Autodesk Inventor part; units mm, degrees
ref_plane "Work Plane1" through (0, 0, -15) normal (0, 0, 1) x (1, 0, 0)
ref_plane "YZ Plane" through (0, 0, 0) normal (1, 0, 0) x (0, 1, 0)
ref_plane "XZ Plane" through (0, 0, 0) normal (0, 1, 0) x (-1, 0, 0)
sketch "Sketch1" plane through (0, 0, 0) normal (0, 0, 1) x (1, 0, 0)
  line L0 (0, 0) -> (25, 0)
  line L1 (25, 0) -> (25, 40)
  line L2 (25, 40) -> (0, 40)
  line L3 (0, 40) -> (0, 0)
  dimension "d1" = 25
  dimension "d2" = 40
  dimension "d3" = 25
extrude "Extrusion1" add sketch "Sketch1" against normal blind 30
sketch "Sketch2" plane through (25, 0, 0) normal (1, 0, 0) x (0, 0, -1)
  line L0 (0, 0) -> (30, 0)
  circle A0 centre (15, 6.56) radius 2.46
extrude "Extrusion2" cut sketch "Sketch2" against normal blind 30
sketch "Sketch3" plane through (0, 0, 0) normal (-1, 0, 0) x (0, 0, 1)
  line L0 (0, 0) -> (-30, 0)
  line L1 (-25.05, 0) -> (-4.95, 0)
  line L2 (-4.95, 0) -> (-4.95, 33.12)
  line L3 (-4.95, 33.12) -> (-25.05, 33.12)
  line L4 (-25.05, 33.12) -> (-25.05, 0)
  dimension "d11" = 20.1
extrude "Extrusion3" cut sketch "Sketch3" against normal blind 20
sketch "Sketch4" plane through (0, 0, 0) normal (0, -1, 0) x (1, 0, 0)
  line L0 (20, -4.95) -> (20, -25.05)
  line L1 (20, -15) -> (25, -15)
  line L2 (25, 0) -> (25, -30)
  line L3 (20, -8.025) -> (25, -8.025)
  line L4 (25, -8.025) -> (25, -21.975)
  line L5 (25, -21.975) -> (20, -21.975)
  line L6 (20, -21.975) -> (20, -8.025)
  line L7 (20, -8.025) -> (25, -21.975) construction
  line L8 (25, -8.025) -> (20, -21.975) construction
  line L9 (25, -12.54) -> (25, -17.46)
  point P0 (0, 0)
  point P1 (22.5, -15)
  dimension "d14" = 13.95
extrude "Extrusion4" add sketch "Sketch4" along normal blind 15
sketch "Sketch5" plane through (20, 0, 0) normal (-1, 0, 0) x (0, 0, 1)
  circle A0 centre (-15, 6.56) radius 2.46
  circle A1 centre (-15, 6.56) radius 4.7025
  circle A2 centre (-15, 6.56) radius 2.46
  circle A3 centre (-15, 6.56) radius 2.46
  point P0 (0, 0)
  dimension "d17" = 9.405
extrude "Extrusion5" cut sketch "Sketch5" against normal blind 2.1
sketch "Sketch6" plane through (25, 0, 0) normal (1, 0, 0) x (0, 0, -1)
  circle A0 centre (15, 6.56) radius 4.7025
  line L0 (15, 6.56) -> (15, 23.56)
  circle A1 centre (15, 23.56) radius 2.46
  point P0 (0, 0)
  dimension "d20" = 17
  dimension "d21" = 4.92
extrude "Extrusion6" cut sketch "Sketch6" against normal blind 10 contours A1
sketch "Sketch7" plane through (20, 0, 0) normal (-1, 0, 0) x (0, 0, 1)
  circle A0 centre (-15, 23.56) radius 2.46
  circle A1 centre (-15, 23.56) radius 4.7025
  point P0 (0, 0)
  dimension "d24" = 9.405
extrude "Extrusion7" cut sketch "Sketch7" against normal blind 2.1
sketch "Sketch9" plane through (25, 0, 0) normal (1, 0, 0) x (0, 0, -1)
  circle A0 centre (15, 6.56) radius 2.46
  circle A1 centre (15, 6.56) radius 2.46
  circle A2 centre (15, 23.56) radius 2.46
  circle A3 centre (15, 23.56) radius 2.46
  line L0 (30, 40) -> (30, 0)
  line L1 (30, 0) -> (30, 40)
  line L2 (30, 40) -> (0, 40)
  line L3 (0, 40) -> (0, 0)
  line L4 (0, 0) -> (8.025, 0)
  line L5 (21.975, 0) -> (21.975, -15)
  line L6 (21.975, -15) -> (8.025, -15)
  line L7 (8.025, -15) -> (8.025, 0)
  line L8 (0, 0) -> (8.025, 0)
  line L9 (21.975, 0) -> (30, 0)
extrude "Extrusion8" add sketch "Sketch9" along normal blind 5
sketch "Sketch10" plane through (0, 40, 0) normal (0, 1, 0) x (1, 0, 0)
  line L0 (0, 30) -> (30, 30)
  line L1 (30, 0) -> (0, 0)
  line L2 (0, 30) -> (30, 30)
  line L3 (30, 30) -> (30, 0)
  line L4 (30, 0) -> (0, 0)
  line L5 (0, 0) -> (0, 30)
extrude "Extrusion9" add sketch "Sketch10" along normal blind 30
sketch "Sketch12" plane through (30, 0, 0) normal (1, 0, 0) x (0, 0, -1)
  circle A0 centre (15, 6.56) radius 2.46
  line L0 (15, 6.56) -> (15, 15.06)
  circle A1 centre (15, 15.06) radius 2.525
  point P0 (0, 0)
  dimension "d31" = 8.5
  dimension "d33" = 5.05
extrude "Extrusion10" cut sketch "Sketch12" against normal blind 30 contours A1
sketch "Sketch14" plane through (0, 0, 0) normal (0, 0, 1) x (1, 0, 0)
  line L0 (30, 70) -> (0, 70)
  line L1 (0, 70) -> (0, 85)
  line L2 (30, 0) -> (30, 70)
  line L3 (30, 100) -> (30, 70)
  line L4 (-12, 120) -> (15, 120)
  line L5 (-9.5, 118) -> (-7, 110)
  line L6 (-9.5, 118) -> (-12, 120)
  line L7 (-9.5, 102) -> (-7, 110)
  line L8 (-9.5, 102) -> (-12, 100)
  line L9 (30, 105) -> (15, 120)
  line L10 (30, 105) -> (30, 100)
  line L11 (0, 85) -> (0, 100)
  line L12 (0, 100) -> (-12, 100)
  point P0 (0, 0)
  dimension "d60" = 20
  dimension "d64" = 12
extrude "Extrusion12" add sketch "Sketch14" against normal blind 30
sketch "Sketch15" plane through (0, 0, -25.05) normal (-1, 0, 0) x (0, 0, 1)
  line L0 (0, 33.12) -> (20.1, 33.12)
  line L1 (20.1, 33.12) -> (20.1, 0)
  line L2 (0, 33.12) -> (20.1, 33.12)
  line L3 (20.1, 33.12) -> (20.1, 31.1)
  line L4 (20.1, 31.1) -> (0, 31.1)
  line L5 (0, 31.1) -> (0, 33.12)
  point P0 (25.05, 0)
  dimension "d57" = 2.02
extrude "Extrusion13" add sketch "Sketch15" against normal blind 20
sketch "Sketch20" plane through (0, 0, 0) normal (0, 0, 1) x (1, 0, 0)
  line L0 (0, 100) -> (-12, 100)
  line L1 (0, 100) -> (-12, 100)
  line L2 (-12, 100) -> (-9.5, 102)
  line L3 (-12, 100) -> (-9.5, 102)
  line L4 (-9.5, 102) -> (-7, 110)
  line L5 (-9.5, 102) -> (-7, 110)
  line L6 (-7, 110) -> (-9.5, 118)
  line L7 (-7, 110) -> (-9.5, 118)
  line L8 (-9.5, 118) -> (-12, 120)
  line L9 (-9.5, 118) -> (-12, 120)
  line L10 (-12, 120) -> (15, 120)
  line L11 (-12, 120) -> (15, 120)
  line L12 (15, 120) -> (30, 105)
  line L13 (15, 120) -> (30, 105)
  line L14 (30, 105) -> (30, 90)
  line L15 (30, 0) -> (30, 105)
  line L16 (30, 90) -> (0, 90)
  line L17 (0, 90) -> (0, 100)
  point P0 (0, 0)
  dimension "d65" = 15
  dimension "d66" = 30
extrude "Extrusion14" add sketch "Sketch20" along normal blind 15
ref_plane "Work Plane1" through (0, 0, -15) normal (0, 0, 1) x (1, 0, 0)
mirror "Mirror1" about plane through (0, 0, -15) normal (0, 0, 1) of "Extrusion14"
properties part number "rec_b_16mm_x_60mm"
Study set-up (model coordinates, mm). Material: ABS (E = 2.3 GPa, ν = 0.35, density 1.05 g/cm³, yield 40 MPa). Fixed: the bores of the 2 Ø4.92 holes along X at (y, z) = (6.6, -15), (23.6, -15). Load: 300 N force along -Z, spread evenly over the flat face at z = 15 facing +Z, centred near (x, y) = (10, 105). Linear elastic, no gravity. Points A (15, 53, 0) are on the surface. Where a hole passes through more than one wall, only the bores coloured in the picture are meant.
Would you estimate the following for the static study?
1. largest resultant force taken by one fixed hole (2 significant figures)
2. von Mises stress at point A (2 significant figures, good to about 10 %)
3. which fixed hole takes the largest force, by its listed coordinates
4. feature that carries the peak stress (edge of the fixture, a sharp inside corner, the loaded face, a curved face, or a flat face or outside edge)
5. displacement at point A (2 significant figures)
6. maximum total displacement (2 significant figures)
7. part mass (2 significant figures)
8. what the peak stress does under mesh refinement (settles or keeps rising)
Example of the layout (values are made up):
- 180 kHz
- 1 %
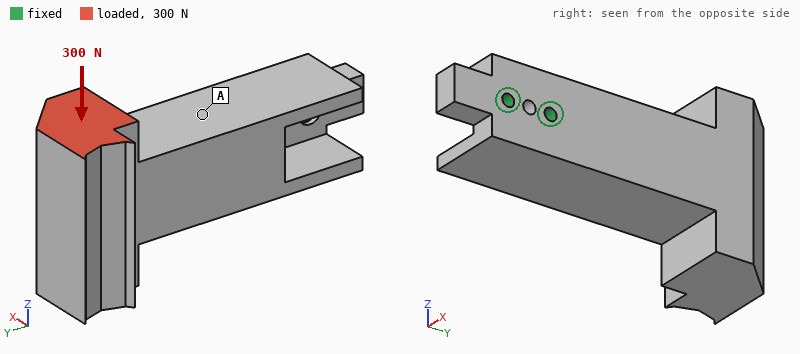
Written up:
- 1.3 kN
- 3.6 MPa
- (23.6, -15)
- edge of the fixture
- 0.45 mm
- 1.6 mm
- 130 g
- keeps rising
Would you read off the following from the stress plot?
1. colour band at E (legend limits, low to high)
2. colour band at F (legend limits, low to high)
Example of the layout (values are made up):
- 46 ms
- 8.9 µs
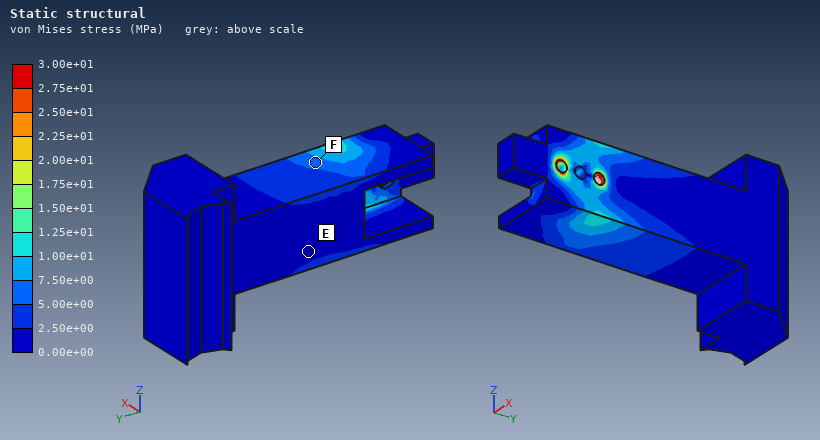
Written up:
- 0.00e+00 to 2.50e+00 MPa
- 5.00e+00 to 7.50e+00 MPa
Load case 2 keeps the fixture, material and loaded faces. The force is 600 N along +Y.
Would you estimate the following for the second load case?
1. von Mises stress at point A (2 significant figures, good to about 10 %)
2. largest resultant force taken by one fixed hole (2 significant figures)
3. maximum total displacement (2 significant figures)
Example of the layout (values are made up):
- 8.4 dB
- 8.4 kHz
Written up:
- 4.7 MPa
- 930 N
- 1.6 mm
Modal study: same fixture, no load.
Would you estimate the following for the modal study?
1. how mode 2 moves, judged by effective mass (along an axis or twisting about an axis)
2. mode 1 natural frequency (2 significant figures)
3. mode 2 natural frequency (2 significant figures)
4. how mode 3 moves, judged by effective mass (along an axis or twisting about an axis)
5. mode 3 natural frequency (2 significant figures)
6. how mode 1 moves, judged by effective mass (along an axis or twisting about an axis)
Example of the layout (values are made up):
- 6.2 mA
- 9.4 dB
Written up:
- along Z
- 240 Hz
- 280 Hz
- twisting about Y
- 620 Hz
- along X
